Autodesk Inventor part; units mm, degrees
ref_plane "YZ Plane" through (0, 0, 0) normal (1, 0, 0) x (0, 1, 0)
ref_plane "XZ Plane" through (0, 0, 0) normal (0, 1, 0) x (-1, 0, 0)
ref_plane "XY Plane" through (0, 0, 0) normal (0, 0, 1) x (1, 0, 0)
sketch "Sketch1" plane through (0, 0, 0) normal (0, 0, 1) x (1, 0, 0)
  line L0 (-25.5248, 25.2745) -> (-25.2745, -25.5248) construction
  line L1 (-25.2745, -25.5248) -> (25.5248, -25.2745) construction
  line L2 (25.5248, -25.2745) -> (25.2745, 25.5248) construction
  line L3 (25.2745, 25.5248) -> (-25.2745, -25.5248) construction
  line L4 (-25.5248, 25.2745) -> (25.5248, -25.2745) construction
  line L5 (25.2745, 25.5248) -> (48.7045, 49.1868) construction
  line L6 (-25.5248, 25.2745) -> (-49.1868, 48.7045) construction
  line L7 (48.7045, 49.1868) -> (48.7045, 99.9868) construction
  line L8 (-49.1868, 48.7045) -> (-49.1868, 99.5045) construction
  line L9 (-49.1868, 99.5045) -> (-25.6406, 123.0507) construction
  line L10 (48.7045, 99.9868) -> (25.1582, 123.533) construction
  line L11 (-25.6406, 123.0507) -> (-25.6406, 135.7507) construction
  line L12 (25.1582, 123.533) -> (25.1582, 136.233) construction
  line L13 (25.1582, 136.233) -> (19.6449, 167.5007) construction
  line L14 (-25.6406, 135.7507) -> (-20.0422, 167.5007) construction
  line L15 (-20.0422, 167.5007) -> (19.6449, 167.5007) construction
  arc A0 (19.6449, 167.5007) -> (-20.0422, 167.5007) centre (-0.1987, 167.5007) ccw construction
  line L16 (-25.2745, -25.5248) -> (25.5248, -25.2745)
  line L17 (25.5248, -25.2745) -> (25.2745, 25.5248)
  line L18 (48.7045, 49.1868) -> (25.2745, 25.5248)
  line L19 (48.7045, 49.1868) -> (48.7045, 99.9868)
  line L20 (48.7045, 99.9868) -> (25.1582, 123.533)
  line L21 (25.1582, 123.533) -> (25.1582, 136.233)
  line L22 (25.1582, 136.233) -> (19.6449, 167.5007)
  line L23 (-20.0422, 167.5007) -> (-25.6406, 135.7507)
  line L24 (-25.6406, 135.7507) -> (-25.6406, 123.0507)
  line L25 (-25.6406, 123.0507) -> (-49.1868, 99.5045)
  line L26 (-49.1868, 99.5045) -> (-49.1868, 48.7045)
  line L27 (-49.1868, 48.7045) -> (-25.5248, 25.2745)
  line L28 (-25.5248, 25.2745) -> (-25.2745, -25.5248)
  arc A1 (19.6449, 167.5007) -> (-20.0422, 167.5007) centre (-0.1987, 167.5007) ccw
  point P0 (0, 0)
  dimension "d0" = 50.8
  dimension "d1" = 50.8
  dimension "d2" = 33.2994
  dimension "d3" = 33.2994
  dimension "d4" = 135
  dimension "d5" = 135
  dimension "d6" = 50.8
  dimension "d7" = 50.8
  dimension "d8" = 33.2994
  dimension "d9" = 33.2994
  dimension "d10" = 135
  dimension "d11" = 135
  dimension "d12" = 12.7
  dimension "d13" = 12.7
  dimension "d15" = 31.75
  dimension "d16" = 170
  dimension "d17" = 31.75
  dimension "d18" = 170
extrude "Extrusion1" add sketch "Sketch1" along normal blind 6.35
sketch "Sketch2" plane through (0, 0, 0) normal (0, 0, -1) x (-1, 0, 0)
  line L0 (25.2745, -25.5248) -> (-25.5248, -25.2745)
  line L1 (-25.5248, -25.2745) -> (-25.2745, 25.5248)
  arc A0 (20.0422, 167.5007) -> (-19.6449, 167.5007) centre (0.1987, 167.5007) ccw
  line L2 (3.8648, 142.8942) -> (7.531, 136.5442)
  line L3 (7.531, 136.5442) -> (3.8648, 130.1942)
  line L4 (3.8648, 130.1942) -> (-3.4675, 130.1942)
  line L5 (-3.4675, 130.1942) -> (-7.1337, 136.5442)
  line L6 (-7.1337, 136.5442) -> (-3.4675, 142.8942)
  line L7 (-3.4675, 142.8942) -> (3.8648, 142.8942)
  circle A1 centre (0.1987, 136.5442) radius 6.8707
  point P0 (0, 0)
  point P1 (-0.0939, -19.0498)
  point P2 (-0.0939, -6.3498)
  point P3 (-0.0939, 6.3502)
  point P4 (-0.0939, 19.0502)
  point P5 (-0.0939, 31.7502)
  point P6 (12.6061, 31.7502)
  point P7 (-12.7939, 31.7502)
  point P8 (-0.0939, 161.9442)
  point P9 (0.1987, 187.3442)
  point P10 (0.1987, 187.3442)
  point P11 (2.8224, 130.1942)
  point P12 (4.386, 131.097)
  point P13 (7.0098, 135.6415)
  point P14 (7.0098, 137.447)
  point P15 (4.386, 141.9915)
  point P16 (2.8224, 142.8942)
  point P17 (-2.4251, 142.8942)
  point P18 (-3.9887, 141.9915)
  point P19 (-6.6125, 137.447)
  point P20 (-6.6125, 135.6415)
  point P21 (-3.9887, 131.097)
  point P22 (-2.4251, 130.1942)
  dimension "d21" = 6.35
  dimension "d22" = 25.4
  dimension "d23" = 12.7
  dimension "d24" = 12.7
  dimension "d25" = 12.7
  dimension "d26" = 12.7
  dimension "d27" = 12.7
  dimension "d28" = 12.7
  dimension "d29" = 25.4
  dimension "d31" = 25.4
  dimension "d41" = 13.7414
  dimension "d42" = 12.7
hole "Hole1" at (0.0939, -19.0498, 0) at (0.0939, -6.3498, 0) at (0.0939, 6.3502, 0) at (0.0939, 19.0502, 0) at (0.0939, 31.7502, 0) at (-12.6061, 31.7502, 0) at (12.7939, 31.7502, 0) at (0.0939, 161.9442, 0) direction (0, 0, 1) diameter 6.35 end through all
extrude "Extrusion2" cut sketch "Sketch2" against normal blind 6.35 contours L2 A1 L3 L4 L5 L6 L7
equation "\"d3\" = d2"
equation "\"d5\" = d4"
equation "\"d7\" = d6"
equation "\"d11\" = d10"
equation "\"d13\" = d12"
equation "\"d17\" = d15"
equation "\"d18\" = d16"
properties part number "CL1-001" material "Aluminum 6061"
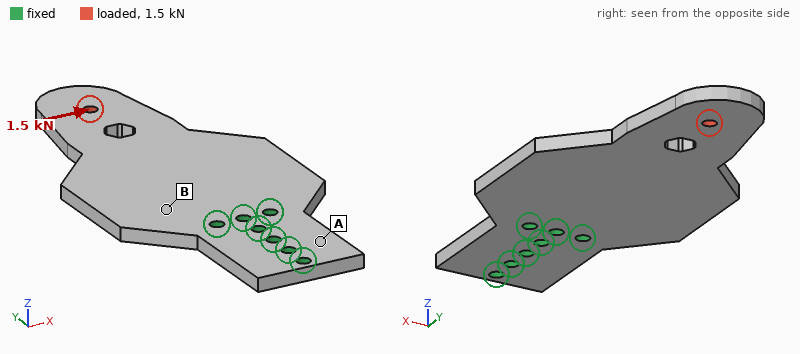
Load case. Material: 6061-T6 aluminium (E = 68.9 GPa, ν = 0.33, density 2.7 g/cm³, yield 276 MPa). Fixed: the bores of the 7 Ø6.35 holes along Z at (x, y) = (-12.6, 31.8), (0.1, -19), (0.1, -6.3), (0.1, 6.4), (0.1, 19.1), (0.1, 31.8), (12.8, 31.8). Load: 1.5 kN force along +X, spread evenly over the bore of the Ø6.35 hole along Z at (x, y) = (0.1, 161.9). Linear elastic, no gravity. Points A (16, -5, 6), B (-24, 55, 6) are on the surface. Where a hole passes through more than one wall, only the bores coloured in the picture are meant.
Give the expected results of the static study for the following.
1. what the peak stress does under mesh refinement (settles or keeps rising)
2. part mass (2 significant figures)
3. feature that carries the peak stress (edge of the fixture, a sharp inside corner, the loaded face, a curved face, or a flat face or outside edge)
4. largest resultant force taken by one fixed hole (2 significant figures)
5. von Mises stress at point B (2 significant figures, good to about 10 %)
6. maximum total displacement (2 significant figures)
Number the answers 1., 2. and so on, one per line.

1. keeps rising
2. 230 g
3. edge of the fixture
4. 4.4 kN
5. 18 MPa
6. 0.19 mm
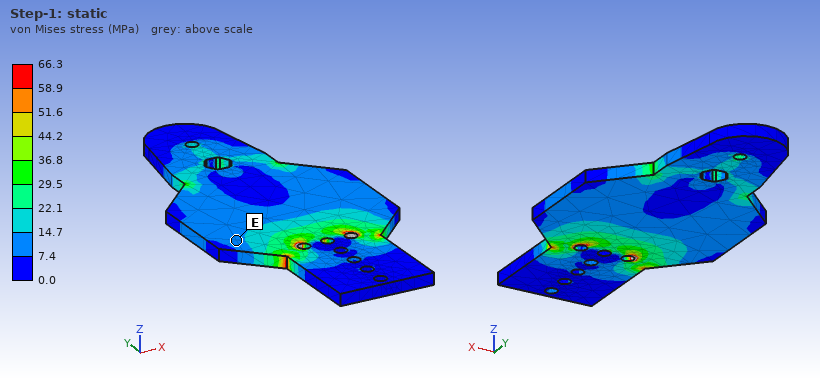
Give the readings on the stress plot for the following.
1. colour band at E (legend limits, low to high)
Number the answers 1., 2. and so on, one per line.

1. 7.4 to 14.7 MPa
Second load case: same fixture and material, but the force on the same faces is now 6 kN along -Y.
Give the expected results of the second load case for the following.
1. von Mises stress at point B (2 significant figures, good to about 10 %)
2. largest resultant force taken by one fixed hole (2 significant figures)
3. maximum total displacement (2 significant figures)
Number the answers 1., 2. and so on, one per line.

1. 12 MPa
2. 2.1 kN
3. 41 µm
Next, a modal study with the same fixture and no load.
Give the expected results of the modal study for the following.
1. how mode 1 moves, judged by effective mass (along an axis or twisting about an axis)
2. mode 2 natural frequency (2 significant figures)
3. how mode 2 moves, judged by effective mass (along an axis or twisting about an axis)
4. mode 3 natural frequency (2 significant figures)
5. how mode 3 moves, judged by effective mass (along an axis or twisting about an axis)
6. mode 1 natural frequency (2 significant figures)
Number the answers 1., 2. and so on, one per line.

1. along Z
2. 1200 Hz
3. twisting about Y
4. 1300 Hz
5. along Z
6. 310 Hz
